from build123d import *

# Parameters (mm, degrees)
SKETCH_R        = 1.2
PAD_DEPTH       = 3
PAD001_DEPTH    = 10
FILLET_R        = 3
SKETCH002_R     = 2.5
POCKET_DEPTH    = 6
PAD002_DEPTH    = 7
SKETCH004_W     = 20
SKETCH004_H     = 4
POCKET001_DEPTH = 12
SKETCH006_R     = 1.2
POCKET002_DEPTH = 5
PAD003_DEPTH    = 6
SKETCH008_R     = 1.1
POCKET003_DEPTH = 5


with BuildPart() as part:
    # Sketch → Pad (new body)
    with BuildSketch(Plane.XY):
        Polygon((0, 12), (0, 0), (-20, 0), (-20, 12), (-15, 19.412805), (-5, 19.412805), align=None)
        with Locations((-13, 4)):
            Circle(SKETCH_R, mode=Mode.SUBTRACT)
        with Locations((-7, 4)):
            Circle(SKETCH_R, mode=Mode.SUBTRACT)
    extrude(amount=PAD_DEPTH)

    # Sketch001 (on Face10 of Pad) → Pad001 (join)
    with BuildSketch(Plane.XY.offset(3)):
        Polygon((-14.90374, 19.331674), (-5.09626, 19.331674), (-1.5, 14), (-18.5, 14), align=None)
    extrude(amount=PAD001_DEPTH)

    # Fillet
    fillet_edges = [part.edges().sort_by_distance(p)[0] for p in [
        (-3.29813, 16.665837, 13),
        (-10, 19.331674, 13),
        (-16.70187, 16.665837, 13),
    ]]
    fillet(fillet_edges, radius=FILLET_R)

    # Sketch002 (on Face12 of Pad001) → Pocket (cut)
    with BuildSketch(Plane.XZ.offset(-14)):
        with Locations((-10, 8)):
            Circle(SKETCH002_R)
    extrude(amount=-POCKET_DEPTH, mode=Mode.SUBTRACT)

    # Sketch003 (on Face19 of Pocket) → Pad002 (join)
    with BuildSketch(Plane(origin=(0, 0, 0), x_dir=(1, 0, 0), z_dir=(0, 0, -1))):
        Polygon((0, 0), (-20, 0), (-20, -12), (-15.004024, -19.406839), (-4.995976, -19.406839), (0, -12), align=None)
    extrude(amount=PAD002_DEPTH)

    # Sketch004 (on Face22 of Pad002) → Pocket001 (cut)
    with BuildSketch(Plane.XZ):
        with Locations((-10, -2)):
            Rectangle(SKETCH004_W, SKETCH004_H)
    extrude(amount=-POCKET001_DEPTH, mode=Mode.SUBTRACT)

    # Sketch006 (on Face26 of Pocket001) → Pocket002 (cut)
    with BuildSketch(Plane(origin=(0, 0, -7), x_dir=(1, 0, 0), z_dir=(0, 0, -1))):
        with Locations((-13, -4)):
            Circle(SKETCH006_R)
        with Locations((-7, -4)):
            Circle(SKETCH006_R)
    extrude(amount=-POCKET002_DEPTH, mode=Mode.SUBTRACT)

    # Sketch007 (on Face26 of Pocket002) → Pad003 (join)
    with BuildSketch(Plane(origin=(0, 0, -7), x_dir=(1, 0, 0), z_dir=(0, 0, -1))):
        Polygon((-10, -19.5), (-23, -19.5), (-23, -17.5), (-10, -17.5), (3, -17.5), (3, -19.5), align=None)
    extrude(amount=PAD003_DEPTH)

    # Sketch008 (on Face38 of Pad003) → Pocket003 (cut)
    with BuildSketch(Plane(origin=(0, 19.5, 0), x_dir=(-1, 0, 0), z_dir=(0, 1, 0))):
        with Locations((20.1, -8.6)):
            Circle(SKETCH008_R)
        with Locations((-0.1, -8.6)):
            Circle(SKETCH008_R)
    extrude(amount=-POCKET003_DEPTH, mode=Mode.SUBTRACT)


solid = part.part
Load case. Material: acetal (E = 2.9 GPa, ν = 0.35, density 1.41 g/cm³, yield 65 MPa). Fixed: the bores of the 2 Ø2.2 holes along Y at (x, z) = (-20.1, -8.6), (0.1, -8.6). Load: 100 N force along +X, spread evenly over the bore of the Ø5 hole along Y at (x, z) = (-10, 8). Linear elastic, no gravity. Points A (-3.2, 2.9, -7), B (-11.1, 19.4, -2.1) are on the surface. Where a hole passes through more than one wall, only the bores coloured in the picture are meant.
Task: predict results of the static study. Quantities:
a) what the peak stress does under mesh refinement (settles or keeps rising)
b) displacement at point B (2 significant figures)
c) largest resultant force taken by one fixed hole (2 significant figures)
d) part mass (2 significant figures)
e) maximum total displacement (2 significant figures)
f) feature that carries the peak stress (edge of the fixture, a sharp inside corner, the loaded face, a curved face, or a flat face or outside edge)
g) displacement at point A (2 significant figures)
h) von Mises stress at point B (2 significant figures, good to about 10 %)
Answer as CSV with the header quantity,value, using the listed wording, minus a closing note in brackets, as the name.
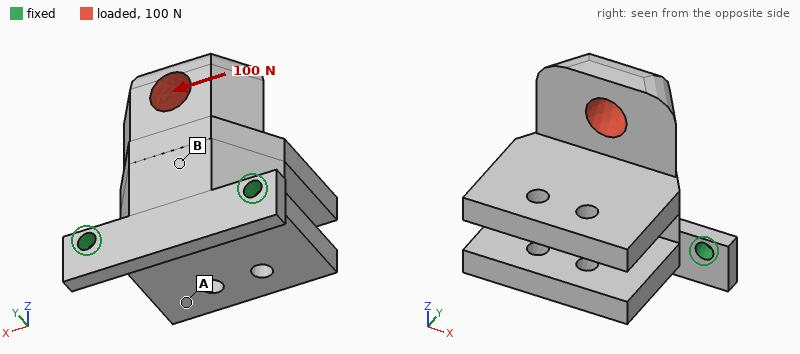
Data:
quantity,value
what the peak stress does under mesh refinement,keeps rising
displacement at point B,0.12 mm
largest resultant force taken by one fixed hole,110 N
part mass,4.7 g
maximum total displacement,0.42 mm
feature that carries the peak stress,a sharp inside corner
displacement at point A,0.14 mm
von Mises stress at point B,8.3 MPa
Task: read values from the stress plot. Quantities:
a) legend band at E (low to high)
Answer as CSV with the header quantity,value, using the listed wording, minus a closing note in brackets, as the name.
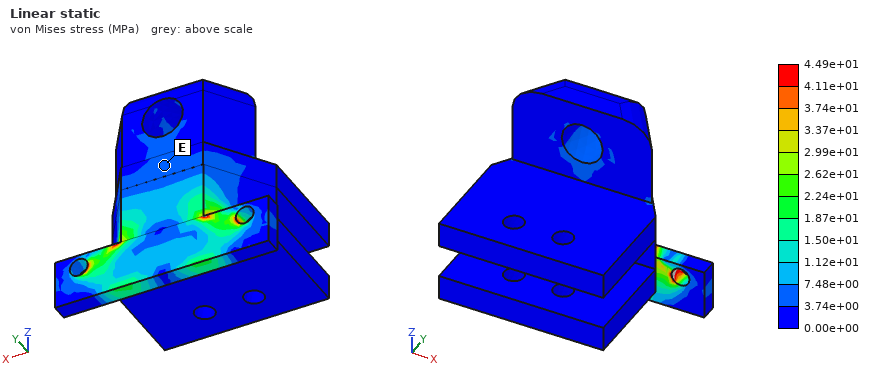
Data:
quantity,value
legend band at E,3.74e+00 to 7.48e+00 MPa
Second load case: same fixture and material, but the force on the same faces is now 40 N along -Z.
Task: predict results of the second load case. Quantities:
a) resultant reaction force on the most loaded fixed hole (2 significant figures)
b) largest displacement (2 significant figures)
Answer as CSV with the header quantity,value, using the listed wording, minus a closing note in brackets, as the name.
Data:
quantity,value
resultant reaction force on the most loaded fixed hole,20 N
largest displacement,0.46 mm
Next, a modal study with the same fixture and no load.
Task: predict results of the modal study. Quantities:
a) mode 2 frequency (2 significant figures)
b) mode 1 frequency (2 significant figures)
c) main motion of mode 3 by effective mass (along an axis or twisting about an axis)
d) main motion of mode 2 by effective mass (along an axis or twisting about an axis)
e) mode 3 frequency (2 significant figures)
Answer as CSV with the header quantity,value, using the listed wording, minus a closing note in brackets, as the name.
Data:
quantity,value
mode 2 frequency,1400 Hz
mode 1 frequency,340 Hz
main motion of mode 3 by effective mass,along X
main motion of mode 2 by effective mass,along X
mode 3 frequency,2200 Hz
